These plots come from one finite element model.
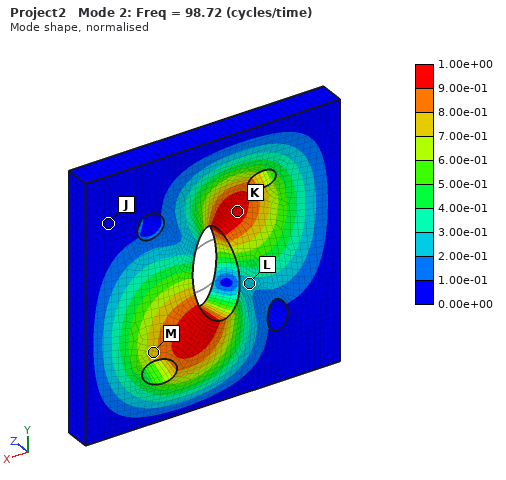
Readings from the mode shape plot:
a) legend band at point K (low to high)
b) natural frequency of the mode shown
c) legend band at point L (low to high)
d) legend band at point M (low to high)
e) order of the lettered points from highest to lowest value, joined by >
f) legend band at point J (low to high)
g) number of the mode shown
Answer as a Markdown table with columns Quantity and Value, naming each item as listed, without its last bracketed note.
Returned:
| Quantity | Value |
|---|---|
| legend band at point K | 9.00e-01 to 1.00e+00 |
| natural frequency of the mode shown | 98.72 |
| legend band at point L | 2.00e-01 to 3.00e-01 |
| legend band at point M | 7.00e-01 to 8.00e-01 |
| order of the lettered points from highest to lowest value, joined by > | K > M > L > J |
| legend band at point J | 0.00e+00 to 1.00e-01 |
| number of the mode shown | 2 |
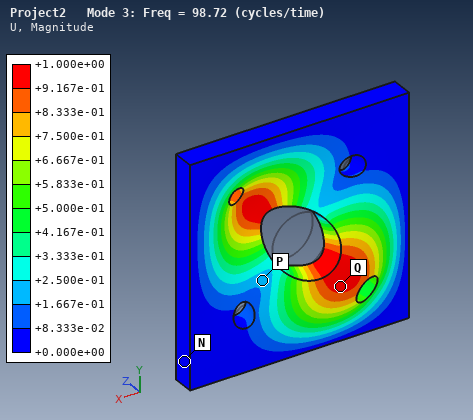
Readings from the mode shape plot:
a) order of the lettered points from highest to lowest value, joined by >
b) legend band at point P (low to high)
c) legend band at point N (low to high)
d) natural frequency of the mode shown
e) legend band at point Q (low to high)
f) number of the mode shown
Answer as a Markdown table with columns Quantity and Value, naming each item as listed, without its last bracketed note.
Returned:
| Quantity | Value |
|---|---|
| order of the lettered points from highest to lowest value, joined by > | Q > P > N |
| legend band at point P | +1.667e-01 to +2.500e-01 |
| legend band at point N | +0.000e+00 to +8.333e-02 |
| natural frequency of the mode shown | 98.72 |
| legend band at point Q | +9.167e-01 to +1.000e+00 |
| number of the mode shown | 3 |
